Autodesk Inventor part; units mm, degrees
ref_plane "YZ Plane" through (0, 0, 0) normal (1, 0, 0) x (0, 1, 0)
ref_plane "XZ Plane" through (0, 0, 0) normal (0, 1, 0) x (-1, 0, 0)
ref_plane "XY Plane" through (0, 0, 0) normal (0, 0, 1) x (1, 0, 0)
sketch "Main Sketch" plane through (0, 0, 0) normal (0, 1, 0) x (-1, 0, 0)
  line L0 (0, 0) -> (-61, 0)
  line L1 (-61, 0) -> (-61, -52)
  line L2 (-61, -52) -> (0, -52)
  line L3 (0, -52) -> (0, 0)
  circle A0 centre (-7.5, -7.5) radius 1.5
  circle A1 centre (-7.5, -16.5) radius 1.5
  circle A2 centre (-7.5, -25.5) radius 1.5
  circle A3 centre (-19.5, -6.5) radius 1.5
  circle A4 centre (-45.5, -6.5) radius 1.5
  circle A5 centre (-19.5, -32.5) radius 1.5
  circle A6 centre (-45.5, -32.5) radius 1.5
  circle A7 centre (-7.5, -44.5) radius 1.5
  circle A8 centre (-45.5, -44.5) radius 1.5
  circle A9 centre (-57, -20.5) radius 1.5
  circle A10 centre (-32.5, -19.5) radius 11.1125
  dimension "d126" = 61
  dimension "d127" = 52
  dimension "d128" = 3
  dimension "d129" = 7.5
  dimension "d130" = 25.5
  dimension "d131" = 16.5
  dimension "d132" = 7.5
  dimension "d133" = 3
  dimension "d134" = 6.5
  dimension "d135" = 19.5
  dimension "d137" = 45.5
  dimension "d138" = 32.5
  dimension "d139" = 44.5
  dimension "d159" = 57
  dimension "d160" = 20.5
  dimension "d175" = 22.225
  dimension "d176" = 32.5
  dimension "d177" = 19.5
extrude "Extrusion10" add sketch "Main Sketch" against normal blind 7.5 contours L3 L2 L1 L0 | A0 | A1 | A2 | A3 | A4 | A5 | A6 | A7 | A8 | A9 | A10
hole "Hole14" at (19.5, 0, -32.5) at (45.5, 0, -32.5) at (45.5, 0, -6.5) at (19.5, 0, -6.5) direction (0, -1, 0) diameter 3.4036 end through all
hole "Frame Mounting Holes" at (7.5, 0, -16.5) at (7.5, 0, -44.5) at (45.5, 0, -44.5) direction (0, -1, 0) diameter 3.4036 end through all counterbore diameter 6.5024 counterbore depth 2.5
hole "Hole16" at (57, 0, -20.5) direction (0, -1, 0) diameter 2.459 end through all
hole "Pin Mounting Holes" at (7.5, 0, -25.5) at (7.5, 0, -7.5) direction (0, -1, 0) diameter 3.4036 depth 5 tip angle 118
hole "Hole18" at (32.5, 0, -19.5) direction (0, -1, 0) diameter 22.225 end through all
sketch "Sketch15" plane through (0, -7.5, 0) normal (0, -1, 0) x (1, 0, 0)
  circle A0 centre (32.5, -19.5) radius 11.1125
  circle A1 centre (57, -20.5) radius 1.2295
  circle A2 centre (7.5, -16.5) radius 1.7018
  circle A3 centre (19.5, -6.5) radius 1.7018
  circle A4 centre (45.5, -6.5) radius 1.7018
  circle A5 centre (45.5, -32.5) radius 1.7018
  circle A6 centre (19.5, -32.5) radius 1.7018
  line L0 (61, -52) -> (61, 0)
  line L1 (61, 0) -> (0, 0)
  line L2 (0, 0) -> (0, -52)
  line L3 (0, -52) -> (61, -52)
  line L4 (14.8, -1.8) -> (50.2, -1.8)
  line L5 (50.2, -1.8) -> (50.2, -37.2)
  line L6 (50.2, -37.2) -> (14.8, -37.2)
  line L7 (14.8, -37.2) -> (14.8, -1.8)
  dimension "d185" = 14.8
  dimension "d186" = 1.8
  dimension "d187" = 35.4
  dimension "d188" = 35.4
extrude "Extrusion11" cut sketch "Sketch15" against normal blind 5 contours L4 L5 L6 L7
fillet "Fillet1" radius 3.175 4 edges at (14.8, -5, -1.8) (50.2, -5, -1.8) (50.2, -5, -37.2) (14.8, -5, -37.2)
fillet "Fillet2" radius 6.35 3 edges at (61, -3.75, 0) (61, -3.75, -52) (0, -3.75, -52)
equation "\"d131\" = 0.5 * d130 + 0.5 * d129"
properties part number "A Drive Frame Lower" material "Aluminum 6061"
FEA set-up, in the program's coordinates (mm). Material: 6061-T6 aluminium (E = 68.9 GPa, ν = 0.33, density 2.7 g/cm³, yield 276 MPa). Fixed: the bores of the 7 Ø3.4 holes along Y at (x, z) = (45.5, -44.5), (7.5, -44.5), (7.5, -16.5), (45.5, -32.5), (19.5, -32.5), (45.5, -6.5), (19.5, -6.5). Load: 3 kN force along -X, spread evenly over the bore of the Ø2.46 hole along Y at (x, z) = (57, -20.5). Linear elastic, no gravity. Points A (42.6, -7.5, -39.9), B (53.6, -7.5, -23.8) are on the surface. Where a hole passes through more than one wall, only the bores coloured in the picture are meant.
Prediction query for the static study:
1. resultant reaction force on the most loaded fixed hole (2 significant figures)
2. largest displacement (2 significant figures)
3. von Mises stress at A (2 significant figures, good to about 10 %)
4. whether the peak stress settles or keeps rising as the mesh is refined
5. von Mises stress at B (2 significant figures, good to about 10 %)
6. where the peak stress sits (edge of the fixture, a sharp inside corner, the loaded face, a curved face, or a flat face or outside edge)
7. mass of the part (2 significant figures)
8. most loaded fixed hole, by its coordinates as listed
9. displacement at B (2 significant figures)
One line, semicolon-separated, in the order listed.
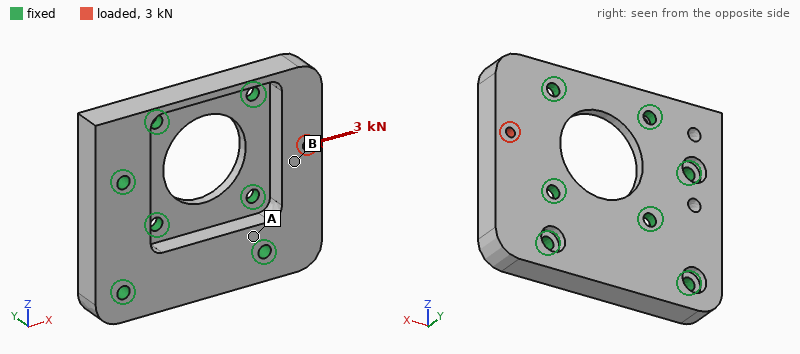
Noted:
1.6 kN; 51 µm; 19 MPa; keeps rising; 50 MPa; edge of the fixture; 43 g; (45.5, -6.5); 32 µm
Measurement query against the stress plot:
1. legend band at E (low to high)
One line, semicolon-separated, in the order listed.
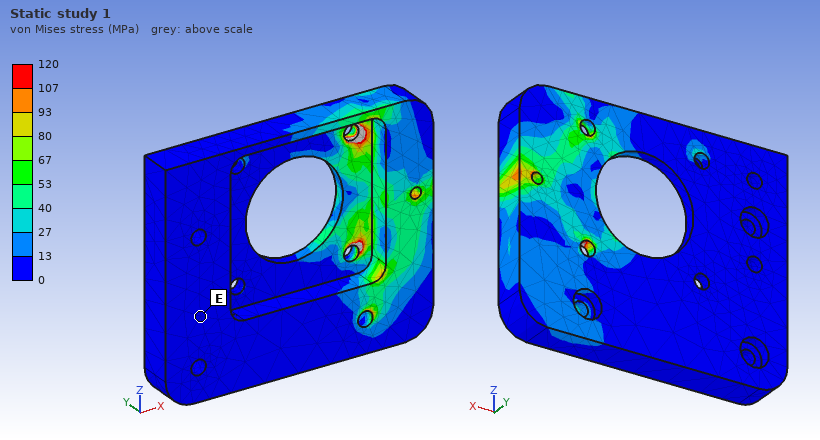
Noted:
0 to 13 MPa
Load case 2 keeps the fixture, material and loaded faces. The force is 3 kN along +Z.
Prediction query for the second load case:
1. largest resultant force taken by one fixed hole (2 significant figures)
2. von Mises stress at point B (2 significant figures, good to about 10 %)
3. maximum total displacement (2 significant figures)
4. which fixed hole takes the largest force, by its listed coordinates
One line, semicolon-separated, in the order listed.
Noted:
1.3 kN; 28 MPa; 14 µm; (45.5, -6.5)
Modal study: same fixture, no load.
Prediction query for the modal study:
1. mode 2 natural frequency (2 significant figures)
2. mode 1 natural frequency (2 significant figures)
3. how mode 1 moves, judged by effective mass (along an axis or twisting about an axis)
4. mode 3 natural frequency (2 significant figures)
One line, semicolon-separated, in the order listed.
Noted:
17 kHz; 9600 Hz; along Y; 19 kHz
